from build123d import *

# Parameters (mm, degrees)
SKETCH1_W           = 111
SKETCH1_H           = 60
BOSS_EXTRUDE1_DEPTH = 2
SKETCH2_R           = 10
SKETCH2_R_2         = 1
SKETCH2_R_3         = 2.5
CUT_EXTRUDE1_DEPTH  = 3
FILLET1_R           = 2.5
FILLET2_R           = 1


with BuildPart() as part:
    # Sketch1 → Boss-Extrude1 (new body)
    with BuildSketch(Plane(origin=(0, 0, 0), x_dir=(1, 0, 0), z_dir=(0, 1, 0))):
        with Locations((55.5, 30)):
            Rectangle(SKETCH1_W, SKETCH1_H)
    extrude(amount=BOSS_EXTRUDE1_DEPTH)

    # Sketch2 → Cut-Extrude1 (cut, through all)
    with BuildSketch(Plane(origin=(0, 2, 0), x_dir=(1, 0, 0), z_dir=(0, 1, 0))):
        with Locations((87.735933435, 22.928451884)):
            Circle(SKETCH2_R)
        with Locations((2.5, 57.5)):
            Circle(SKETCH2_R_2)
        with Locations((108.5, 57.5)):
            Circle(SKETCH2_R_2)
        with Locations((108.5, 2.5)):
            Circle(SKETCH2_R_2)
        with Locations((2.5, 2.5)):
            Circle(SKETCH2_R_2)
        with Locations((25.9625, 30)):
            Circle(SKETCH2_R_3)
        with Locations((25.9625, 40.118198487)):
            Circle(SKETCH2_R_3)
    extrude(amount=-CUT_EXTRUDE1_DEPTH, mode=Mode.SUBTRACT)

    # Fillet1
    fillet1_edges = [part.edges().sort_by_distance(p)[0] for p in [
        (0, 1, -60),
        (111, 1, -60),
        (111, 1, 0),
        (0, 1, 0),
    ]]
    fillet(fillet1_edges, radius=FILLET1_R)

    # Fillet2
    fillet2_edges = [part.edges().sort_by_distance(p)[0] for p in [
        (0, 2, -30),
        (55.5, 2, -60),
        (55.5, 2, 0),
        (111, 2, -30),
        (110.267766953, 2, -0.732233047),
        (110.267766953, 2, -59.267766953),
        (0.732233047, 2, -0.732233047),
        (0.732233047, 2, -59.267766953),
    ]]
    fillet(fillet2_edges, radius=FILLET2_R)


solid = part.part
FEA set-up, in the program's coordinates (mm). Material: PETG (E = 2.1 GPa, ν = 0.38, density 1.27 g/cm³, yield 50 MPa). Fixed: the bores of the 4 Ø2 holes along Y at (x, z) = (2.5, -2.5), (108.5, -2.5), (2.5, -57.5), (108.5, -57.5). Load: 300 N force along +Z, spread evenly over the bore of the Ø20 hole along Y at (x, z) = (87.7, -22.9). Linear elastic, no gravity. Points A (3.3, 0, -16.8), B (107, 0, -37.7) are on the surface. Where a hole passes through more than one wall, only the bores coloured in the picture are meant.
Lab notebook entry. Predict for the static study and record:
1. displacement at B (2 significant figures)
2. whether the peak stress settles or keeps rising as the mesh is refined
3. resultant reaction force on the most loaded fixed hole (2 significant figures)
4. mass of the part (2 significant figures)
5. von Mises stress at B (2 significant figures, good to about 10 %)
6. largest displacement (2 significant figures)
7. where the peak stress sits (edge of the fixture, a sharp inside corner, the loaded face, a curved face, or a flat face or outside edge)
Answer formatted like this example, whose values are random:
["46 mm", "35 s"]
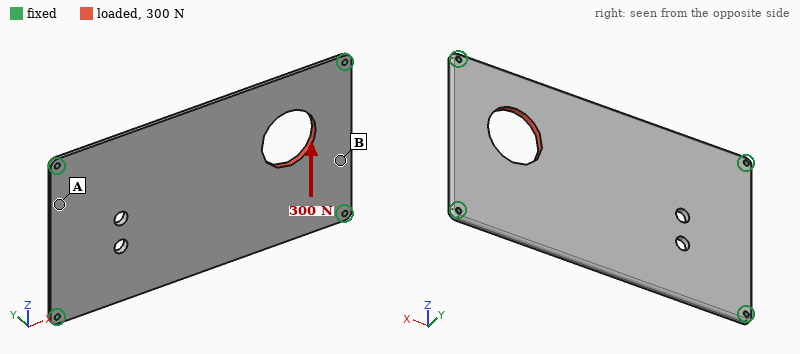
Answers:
["0.055 mm", "keeps rising", "130 N", "16 g", "2.8 MPa", "0.15 mm", "edge of the fixture"]
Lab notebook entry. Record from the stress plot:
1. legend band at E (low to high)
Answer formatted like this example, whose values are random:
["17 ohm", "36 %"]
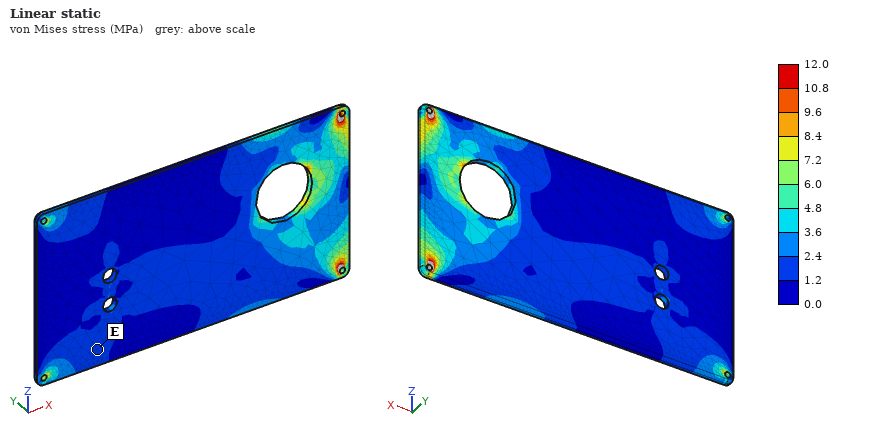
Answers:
["1.2 to 2.4 MPa"]
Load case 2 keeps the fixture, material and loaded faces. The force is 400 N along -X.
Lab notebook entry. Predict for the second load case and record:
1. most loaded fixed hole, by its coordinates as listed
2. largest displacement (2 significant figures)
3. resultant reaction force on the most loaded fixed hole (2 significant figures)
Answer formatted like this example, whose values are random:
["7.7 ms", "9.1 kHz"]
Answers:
["(108.5, -2.5)", "0.14 mm", "160 N"]
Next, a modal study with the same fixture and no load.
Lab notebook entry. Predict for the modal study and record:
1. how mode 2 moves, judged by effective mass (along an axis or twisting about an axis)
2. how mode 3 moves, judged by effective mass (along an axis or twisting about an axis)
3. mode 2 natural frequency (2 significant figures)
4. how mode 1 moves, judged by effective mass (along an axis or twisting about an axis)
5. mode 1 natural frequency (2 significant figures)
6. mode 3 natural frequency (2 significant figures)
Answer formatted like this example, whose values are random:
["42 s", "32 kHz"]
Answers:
["twisting about X", "twisting about Z", "330 Hz", "along Y", "180 Hz", "510 Hz"]
